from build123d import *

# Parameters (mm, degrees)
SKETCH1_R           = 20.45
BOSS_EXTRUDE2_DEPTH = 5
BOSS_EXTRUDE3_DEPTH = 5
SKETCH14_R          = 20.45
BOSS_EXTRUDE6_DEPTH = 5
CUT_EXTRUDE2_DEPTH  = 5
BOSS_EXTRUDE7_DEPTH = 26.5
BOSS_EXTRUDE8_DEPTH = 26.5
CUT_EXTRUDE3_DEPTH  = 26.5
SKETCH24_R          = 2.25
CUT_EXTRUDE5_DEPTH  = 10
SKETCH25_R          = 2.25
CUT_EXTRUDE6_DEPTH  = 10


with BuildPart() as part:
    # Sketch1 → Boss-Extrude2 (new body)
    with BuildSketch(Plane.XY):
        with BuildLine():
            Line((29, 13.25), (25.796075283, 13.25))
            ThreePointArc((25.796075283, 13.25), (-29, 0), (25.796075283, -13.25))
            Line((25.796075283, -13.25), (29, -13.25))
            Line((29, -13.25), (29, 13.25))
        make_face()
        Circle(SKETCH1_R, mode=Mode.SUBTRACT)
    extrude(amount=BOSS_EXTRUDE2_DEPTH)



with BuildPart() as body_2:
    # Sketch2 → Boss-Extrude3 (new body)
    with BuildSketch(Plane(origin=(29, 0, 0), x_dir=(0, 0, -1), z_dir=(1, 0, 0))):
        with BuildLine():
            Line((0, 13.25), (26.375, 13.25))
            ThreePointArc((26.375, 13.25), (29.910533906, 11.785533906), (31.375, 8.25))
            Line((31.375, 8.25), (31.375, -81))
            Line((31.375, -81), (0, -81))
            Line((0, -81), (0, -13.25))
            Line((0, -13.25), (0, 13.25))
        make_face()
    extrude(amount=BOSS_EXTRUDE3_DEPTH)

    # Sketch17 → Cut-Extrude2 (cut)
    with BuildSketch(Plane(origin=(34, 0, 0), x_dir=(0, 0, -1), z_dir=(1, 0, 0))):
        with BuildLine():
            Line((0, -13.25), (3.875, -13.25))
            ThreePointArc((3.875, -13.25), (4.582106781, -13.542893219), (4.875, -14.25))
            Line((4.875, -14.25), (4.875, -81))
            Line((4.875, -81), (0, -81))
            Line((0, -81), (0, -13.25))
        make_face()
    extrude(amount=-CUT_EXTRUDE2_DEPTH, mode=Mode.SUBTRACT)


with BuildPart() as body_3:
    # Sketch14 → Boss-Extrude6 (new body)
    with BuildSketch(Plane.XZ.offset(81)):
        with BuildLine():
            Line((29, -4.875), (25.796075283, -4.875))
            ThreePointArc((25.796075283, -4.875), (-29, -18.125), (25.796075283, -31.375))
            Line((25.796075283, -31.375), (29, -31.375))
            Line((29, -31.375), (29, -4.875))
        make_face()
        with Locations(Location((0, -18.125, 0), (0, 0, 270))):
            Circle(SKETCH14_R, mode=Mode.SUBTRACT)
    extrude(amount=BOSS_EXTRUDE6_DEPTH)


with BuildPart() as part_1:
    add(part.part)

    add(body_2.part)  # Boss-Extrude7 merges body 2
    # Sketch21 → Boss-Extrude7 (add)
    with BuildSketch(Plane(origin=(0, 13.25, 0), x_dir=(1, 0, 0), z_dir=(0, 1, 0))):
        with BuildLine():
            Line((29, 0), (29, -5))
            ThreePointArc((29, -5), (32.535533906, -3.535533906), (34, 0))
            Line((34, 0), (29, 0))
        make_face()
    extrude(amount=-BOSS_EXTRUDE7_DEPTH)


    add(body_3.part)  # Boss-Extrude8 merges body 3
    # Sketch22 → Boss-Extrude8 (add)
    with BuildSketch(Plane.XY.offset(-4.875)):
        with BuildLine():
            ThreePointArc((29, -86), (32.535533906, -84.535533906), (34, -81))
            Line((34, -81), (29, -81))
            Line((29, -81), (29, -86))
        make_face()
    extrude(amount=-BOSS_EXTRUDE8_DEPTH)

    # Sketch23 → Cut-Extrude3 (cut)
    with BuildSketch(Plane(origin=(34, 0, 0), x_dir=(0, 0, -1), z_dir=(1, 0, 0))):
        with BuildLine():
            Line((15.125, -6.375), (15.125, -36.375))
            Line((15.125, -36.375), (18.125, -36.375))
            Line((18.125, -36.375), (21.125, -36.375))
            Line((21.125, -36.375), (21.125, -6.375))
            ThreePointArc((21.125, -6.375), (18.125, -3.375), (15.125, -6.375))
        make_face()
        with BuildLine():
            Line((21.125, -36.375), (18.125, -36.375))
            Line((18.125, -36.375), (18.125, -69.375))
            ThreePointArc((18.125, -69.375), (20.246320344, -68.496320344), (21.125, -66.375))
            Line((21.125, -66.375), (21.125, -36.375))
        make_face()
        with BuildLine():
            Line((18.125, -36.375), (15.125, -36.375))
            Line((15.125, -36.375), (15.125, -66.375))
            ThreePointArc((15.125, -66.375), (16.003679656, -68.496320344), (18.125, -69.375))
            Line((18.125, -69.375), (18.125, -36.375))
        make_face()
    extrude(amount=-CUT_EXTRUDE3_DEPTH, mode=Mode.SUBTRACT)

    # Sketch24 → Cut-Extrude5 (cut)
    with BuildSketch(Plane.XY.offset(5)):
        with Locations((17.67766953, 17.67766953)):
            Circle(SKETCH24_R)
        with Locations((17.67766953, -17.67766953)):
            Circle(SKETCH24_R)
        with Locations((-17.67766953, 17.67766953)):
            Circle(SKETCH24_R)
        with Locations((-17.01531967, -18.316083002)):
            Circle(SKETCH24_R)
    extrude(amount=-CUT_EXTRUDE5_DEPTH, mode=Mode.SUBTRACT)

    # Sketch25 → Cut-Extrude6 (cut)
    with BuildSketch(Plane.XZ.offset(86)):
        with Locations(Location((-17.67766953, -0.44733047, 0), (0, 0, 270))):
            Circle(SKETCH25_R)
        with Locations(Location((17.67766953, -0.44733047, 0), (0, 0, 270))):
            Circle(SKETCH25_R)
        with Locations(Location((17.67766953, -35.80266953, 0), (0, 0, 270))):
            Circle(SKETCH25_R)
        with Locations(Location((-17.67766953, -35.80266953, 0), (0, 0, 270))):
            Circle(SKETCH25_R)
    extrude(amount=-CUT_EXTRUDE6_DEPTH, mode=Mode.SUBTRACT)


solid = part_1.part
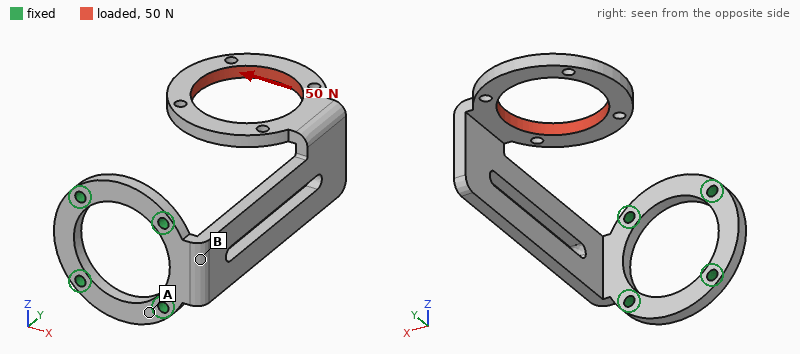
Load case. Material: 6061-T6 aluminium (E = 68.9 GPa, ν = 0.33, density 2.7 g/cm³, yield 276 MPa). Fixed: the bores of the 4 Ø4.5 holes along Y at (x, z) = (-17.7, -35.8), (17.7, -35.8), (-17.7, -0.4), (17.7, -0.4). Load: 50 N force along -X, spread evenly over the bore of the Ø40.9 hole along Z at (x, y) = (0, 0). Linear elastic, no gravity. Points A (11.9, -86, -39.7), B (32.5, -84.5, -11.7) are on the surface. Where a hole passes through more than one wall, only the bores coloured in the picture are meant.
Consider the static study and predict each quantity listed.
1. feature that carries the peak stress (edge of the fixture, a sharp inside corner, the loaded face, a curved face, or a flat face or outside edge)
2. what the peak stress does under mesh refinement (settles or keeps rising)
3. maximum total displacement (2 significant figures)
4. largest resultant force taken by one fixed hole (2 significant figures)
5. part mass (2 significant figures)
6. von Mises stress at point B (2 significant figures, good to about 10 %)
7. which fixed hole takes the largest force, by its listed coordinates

edge of the fixture
keeps rising
1.6 mm
76 N
68 g
19 MPa
(17.7, -0.4)
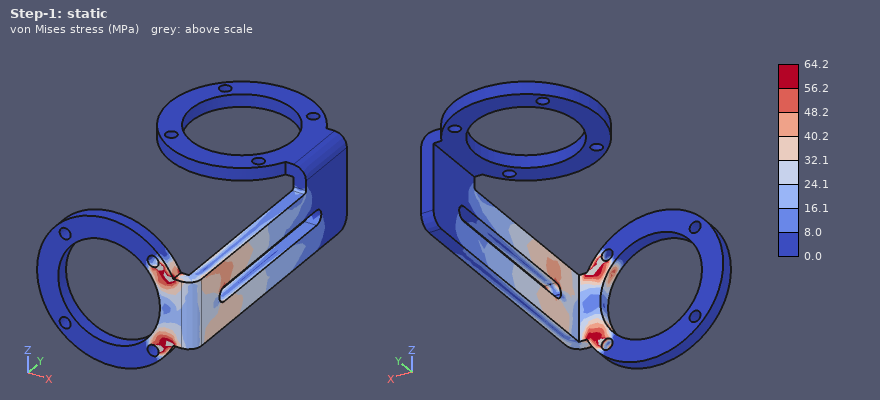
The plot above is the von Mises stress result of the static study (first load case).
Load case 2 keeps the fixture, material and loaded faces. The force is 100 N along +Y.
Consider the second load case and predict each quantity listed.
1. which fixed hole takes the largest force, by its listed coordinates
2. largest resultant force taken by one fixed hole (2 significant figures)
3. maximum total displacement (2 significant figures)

(17.7, -0.4)
120 N
1.7 mm
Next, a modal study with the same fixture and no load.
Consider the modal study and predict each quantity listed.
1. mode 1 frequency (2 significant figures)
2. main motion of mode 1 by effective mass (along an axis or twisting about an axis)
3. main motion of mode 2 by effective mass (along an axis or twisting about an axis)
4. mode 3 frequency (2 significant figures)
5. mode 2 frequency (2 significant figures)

180 Hz
along X
along Z
690 Hz
350 Hz
